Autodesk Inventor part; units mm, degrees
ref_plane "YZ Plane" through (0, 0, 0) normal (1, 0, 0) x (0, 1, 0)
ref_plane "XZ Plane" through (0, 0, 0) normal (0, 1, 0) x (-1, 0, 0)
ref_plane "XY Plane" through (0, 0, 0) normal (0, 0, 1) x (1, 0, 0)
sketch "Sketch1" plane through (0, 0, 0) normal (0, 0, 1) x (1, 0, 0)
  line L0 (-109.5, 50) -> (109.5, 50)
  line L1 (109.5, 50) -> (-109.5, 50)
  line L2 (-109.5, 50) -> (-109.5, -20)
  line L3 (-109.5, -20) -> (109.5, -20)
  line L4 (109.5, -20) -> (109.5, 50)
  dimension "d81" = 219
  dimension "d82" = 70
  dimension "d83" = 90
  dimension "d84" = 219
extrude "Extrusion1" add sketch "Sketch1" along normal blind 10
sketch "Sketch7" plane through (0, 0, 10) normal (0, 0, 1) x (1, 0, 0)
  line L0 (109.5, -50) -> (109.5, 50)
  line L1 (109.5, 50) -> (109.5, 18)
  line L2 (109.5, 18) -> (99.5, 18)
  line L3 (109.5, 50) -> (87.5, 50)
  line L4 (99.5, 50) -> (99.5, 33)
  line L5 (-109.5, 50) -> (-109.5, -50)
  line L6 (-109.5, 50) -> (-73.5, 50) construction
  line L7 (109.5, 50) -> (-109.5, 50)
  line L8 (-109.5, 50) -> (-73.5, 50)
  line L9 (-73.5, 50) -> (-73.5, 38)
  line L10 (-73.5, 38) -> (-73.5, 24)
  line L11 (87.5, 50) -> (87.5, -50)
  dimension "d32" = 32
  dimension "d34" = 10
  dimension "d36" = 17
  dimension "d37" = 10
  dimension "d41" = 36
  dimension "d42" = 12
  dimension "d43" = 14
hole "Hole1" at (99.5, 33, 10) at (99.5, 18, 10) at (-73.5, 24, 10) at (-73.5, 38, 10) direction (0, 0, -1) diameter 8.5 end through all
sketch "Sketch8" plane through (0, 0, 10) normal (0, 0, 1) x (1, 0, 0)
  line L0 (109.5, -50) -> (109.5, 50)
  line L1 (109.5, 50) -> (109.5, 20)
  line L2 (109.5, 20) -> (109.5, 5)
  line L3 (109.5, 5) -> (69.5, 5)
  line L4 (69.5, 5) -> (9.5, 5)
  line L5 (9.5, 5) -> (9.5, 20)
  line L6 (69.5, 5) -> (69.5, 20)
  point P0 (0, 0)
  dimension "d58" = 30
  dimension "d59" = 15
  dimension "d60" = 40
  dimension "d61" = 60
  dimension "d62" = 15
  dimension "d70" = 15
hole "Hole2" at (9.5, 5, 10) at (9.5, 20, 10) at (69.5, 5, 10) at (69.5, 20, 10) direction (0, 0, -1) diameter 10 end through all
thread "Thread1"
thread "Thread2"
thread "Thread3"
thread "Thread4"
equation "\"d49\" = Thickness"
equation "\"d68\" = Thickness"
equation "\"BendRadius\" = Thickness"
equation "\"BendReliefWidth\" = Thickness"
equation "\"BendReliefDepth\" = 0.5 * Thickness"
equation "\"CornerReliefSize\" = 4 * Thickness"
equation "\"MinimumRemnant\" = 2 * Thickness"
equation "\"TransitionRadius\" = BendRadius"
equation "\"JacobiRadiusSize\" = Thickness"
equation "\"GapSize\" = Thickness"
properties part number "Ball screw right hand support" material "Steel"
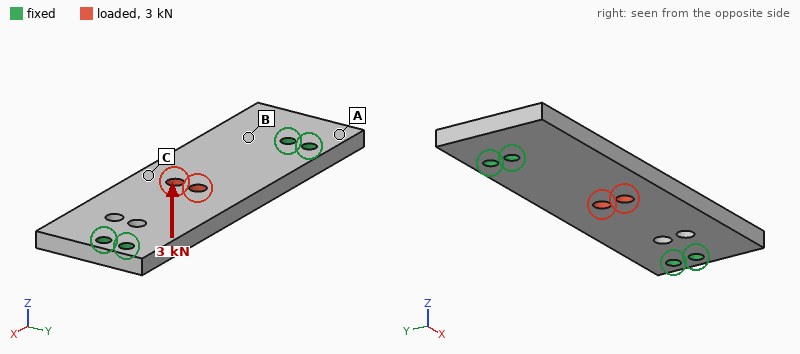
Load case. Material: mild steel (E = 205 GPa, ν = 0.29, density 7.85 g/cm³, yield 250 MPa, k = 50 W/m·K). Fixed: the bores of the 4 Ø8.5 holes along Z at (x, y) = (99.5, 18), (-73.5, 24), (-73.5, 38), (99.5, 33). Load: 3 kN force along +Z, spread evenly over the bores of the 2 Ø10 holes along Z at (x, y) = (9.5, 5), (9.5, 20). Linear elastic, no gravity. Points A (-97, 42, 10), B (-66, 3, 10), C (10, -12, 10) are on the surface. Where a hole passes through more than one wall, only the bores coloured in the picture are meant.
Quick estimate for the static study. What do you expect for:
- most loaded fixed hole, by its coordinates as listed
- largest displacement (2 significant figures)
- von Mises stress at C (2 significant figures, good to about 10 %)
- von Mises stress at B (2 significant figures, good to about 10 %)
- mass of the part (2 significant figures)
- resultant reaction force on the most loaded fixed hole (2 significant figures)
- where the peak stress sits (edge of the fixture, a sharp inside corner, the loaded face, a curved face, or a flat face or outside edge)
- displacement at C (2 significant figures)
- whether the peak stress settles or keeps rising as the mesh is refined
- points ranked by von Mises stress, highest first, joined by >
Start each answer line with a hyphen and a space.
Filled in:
- (-73.5, 24)
- 99 µm
- 60 MPa
- 32 MPa
- 1.2 kg
- 1.6 kN
- edge of the fixture
- 95 µm
- keeps rising
- C > B > A
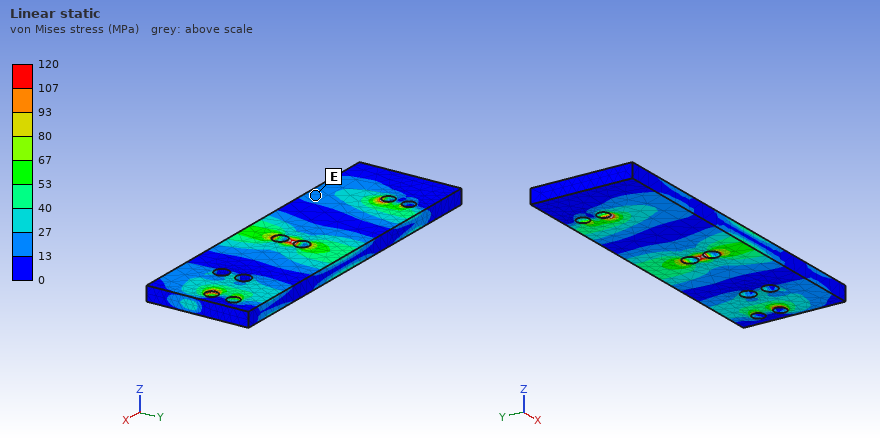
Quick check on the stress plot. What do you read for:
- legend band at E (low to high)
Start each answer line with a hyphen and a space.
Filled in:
- 13 to 27 MPa
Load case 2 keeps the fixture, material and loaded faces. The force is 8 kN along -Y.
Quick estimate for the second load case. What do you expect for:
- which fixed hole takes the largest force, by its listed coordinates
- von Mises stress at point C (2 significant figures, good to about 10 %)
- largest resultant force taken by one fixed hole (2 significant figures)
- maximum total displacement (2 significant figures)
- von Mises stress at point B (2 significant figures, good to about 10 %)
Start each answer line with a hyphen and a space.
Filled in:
- (-73.5, 38)
- 26 MPa
- 5.0 kN
- 17 µm
- 7.0 MPa
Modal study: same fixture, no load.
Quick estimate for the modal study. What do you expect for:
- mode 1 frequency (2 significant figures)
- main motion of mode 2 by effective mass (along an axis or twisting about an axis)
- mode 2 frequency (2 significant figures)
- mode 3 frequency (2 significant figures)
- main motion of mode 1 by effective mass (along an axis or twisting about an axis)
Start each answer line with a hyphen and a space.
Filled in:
- 1600 Hz
- twisting about X
- 2600 Hz
- 3700 Hz
- along Z
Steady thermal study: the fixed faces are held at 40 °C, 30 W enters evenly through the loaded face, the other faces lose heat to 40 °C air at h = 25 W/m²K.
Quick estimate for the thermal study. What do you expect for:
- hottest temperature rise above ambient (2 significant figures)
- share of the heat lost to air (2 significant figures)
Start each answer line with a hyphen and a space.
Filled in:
- 39 K
- 36 %
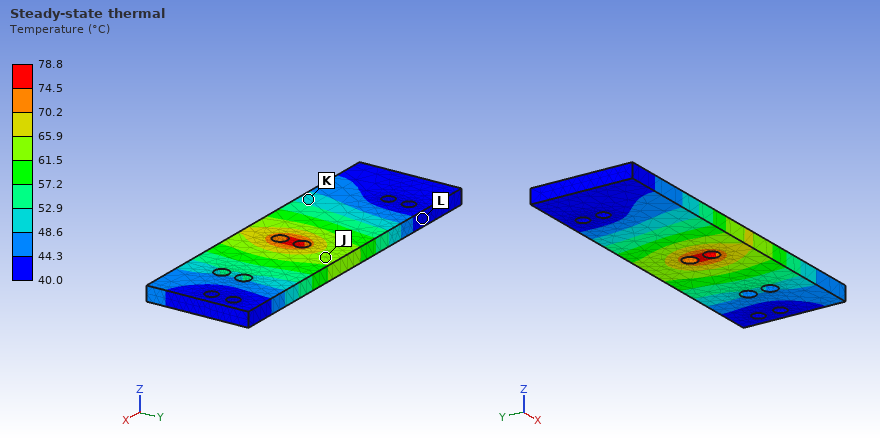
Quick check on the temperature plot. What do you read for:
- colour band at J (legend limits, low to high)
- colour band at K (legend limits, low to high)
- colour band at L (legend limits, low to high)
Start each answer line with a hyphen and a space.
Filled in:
- 61.5 to 65.9 °C
- 48.6 to 52.9 °C
- 40.0 to 44.3 °C
